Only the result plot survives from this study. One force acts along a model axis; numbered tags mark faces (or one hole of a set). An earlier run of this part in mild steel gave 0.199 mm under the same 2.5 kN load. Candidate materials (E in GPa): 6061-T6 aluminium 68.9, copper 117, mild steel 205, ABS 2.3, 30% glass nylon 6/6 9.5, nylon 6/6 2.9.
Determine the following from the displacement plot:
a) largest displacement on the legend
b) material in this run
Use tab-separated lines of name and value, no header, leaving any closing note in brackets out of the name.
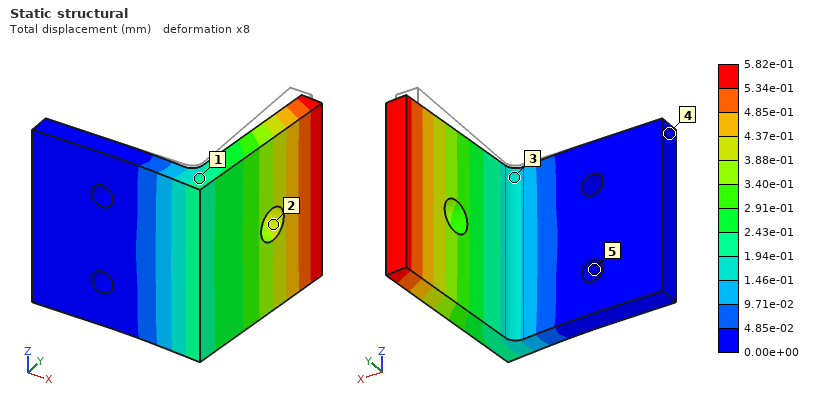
largest displacement on the legend	5.82e-01 mm
material in this run	6061-T6 aluminium
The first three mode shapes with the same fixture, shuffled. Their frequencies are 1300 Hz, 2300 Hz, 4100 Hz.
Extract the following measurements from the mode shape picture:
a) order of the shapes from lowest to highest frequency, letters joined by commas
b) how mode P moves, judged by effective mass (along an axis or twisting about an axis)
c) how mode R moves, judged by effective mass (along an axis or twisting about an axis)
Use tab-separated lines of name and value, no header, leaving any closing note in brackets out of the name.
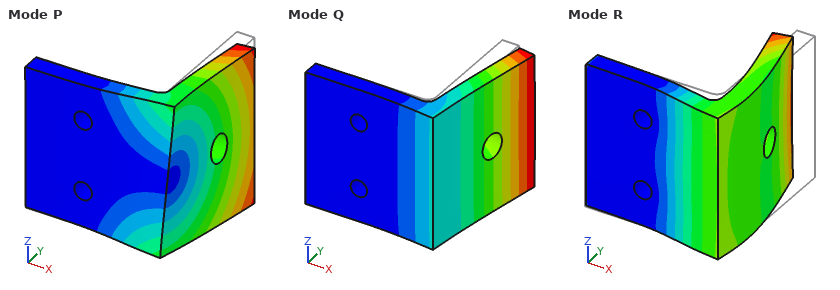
order of the shapes from lowest to highest frequency, letters joined by commas	Q, P, R
how mode P moves, judged by effective mass	along Z
how mode R moves, judged by effective mass	along Y
